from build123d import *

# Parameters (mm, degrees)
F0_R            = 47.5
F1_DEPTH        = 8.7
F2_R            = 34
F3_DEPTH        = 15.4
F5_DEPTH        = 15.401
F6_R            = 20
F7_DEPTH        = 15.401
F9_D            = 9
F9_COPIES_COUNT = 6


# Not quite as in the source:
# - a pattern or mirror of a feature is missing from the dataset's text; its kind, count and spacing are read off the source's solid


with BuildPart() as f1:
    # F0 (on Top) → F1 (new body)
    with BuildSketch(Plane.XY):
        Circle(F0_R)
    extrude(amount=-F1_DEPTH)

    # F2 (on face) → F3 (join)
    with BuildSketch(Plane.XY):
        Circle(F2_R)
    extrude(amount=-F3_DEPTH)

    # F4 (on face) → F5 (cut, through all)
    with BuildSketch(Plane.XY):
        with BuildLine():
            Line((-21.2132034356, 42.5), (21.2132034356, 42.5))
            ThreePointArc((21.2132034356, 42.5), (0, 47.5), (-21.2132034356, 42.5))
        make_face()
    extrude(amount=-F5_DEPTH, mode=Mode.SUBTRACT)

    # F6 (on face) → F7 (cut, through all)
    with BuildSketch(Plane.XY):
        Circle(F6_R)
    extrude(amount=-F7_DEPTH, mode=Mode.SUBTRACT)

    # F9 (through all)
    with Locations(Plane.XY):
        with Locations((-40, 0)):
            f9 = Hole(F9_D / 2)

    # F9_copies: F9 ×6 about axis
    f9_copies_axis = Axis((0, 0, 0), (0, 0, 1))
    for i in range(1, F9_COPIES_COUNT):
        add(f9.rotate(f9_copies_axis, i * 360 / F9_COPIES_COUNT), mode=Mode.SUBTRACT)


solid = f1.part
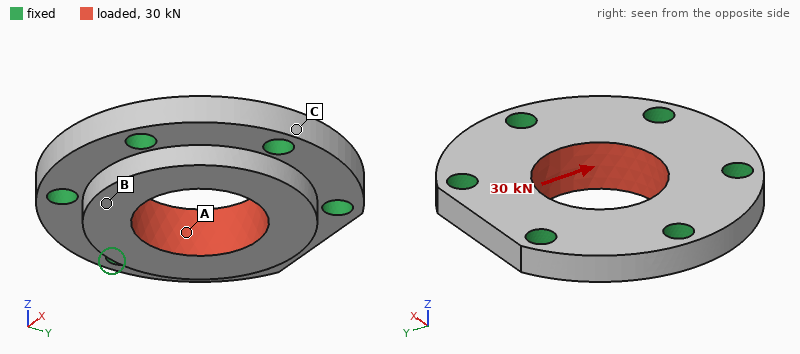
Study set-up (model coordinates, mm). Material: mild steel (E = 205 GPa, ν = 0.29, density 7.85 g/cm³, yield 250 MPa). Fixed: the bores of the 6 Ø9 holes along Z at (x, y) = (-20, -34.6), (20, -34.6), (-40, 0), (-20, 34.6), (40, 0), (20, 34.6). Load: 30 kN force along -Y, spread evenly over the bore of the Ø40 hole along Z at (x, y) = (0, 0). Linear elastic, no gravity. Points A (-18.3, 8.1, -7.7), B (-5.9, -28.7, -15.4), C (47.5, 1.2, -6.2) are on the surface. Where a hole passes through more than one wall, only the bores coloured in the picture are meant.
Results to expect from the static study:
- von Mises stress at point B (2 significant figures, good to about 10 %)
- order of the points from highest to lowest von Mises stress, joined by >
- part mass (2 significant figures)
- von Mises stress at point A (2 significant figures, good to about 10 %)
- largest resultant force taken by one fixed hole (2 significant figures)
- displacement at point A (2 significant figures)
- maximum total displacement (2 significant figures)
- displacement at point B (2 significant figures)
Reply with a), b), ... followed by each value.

a) 15 MPa
b) A > B > C
c) 490 g
d) 30 MPa
e) 6.1 kN
f) 3.1 µm
g) 5.1 µm
h) 3.8 µm
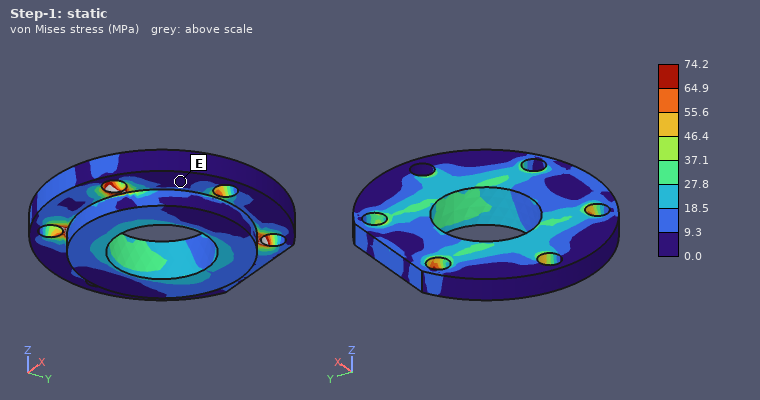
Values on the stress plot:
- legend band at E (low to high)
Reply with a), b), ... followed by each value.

a) 0.0 to 9.3 MPa
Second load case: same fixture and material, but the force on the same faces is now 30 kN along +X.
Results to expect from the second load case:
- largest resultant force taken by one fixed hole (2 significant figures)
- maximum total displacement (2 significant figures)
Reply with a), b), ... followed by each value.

a) 6.7 kN
b) 4.6 µm
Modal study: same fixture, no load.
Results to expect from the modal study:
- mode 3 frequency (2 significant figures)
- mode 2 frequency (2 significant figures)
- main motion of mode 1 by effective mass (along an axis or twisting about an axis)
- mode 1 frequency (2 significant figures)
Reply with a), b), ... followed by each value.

a) 23 kHz
b) 23 kHz
c) along Z
d) 18 kHz
